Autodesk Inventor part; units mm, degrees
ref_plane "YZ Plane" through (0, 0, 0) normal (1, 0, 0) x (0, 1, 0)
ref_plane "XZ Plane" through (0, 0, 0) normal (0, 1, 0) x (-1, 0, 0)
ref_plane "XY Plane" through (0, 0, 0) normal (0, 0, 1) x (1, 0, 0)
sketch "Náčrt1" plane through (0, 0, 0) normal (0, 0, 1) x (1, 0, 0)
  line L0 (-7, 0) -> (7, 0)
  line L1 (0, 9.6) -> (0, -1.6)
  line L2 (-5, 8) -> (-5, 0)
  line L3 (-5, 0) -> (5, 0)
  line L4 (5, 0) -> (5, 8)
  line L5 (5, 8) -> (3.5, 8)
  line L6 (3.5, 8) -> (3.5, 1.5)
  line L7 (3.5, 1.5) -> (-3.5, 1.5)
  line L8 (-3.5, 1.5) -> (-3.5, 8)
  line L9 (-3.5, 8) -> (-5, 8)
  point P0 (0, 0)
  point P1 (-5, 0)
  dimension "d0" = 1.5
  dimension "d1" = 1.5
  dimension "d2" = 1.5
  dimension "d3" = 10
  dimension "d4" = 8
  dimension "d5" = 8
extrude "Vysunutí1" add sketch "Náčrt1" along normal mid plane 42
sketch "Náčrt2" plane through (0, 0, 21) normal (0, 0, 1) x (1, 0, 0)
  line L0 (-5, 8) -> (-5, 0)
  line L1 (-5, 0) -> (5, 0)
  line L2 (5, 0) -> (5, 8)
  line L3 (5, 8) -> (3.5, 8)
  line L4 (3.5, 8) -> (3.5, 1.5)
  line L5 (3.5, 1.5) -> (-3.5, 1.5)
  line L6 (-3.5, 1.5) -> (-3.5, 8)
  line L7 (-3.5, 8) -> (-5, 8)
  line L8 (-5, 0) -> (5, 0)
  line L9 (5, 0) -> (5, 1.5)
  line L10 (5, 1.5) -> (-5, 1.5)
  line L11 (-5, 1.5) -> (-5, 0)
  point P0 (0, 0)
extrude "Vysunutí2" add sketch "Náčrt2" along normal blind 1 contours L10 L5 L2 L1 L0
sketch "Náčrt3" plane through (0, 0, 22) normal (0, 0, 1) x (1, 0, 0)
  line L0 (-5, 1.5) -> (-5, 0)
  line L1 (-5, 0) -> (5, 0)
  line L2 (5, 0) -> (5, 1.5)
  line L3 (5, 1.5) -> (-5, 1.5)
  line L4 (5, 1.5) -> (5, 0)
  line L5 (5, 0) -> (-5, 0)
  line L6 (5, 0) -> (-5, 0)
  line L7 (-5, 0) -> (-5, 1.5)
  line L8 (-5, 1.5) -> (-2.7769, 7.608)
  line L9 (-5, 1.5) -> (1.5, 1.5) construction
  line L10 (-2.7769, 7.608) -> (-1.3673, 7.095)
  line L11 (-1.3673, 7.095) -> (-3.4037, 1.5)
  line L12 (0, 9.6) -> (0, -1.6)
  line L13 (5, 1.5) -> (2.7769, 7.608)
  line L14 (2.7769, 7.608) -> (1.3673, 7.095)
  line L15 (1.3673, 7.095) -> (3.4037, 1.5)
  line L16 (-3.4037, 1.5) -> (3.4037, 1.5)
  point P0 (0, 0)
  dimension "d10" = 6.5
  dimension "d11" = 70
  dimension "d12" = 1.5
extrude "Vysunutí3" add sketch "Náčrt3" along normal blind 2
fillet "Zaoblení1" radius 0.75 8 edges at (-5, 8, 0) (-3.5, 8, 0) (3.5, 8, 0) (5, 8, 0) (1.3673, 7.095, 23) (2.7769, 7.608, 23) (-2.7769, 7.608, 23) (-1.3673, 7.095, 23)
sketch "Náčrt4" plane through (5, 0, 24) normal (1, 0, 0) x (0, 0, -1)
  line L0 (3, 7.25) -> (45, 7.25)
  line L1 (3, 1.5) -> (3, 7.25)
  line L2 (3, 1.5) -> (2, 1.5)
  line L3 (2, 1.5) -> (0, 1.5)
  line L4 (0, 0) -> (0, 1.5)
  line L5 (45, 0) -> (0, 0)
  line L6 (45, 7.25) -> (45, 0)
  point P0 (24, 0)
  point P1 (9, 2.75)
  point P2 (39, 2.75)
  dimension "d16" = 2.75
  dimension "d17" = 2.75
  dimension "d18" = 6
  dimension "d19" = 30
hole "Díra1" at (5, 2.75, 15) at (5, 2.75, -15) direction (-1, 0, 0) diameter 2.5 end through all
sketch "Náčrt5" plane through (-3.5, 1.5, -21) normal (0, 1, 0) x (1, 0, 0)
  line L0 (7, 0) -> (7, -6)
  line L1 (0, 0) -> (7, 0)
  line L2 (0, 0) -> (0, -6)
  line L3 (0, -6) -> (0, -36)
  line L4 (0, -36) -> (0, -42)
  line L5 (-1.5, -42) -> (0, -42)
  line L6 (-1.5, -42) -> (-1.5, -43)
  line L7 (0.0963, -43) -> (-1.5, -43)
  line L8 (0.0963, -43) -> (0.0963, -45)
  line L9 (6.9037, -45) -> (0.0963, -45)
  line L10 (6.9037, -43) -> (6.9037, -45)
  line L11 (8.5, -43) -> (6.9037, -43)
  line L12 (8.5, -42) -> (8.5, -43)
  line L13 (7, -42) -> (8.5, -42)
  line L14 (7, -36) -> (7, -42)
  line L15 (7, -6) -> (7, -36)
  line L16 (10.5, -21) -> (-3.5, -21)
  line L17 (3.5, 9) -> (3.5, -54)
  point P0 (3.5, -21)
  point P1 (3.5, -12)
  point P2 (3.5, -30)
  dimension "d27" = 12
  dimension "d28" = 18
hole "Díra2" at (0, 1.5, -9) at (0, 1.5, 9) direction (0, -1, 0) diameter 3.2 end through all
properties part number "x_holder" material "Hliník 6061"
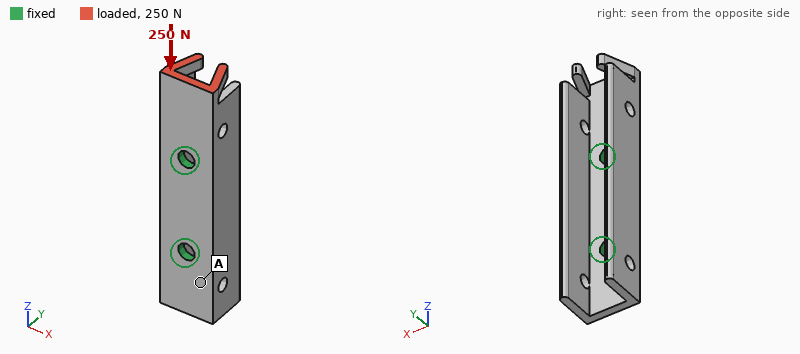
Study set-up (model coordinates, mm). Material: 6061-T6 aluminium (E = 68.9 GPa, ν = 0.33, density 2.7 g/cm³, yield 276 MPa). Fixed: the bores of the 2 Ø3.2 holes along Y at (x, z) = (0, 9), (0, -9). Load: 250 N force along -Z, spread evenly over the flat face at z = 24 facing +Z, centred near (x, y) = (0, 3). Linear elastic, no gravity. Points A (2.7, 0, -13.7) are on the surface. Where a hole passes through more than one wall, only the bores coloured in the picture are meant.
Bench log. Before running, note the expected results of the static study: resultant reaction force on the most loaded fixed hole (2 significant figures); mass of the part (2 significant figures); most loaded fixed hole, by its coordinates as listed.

190 N
3.9 g
(0, 9)
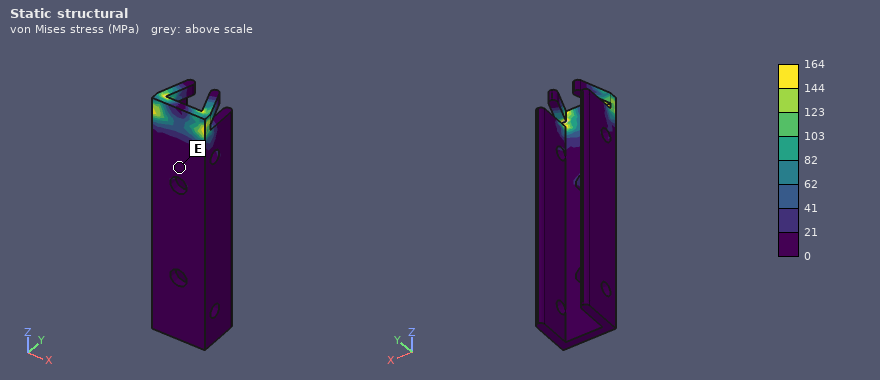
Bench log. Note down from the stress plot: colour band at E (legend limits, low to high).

0 to 21 MPa
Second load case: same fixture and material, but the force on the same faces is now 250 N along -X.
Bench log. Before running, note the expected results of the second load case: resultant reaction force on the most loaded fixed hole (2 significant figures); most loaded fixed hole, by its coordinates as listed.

360 N
(0, 9)
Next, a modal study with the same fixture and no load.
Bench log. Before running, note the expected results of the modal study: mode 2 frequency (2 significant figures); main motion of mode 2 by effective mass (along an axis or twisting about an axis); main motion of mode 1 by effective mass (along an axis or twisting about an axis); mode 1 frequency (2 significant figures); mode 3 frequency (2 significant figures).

11 kHz
along X
along X
10 kHz
13 kHz
